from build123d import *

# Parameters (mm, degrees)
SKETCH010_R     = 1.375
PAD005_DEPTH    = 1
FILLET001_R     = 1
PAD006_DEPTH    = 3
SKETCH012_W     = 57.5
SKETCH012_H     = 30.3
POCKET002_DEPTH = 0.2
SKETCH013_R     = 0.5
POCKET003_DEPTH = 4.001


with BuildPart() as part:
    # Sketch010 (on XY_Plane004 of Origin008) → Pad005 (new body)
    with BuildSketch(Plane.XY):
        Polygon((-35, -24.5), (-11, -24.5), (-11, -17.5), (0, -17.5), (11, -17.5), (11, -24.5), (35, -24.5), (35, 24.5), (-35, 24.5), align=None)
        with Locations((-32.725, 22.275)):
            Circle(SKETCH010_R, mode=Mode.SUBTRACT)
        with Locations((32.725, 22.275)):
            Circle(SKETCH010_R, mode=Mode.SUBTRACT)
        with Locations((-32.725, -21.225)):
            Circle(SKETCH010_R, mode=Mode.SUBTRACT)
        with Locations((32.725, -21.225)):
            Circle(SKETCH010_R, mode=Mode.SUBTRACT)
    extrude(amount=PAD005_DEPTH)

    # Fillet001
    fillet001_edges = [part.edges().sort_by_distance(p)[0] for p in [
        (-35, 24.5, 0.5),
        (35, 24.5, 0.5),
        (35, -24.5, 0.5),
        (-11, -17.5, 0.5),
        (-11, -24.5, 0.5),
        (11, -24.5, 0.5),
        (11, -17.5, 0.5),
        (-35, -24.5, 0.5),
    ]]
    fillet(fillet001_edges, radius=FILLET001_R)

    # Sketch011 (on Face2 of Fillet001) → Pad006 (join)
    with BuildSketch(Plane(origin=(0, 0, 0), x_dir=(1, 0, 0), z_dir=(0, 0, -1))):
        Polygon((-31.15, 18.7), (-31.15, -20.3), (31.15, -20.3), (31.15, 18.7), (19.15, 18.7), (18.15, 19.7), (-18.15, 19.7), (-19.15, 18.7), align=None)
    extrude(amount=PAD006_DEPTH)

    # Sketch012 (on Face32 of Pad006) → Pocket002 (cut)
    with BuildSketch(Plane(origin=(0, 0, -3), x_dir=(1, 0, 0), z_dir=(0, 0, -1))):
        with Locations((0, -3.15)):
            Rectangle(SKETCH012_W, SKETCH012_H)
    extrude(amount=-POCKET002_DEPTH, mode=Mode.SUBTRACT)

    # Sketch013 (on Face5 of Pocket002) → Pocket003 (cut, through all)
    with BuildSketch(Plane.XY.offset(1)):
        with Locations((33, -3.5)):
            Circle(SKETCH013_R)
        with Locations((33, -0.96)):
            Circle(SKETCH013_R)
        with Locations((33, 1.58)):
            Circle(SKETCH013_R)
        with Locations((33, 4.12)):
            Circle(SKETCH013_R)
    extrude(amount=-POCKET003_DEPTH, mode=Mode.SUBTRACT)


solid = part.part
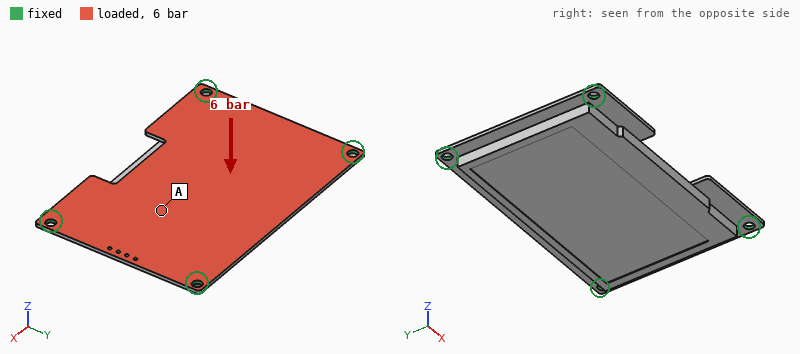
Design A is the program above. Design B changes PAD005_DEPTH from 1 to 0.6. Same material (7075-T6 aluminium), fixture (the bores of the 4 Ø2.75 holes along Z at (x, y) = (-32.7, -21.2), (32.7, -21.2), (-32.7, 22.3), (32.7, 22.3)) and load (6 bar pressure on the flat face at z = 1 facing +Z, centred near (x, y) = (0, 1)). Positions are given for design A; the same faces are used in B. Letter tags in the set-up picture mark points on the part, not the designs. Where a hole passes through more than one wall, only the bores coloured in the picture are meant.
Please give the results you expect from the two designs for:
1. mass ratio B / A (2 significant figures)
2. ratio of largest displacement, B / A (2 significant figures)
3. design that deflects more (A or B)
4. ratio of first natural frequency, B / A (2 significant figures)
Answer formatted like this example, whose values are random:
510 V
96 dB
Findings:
0.87
1.6
B
0.84
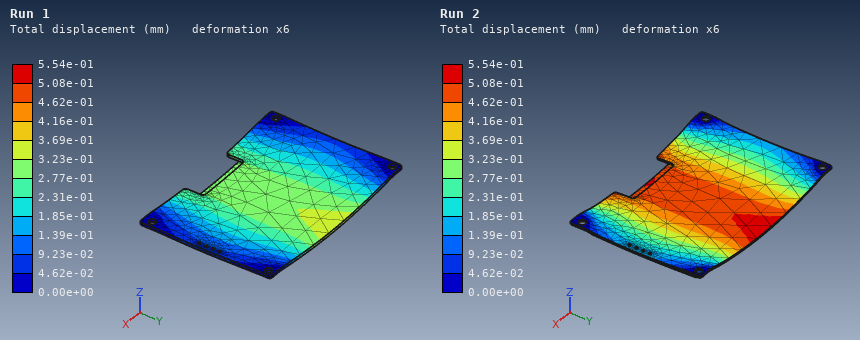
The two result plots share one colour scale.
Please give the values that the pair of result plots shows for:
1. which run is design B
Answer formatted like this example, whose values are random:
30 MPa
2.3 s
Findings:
Run 2
